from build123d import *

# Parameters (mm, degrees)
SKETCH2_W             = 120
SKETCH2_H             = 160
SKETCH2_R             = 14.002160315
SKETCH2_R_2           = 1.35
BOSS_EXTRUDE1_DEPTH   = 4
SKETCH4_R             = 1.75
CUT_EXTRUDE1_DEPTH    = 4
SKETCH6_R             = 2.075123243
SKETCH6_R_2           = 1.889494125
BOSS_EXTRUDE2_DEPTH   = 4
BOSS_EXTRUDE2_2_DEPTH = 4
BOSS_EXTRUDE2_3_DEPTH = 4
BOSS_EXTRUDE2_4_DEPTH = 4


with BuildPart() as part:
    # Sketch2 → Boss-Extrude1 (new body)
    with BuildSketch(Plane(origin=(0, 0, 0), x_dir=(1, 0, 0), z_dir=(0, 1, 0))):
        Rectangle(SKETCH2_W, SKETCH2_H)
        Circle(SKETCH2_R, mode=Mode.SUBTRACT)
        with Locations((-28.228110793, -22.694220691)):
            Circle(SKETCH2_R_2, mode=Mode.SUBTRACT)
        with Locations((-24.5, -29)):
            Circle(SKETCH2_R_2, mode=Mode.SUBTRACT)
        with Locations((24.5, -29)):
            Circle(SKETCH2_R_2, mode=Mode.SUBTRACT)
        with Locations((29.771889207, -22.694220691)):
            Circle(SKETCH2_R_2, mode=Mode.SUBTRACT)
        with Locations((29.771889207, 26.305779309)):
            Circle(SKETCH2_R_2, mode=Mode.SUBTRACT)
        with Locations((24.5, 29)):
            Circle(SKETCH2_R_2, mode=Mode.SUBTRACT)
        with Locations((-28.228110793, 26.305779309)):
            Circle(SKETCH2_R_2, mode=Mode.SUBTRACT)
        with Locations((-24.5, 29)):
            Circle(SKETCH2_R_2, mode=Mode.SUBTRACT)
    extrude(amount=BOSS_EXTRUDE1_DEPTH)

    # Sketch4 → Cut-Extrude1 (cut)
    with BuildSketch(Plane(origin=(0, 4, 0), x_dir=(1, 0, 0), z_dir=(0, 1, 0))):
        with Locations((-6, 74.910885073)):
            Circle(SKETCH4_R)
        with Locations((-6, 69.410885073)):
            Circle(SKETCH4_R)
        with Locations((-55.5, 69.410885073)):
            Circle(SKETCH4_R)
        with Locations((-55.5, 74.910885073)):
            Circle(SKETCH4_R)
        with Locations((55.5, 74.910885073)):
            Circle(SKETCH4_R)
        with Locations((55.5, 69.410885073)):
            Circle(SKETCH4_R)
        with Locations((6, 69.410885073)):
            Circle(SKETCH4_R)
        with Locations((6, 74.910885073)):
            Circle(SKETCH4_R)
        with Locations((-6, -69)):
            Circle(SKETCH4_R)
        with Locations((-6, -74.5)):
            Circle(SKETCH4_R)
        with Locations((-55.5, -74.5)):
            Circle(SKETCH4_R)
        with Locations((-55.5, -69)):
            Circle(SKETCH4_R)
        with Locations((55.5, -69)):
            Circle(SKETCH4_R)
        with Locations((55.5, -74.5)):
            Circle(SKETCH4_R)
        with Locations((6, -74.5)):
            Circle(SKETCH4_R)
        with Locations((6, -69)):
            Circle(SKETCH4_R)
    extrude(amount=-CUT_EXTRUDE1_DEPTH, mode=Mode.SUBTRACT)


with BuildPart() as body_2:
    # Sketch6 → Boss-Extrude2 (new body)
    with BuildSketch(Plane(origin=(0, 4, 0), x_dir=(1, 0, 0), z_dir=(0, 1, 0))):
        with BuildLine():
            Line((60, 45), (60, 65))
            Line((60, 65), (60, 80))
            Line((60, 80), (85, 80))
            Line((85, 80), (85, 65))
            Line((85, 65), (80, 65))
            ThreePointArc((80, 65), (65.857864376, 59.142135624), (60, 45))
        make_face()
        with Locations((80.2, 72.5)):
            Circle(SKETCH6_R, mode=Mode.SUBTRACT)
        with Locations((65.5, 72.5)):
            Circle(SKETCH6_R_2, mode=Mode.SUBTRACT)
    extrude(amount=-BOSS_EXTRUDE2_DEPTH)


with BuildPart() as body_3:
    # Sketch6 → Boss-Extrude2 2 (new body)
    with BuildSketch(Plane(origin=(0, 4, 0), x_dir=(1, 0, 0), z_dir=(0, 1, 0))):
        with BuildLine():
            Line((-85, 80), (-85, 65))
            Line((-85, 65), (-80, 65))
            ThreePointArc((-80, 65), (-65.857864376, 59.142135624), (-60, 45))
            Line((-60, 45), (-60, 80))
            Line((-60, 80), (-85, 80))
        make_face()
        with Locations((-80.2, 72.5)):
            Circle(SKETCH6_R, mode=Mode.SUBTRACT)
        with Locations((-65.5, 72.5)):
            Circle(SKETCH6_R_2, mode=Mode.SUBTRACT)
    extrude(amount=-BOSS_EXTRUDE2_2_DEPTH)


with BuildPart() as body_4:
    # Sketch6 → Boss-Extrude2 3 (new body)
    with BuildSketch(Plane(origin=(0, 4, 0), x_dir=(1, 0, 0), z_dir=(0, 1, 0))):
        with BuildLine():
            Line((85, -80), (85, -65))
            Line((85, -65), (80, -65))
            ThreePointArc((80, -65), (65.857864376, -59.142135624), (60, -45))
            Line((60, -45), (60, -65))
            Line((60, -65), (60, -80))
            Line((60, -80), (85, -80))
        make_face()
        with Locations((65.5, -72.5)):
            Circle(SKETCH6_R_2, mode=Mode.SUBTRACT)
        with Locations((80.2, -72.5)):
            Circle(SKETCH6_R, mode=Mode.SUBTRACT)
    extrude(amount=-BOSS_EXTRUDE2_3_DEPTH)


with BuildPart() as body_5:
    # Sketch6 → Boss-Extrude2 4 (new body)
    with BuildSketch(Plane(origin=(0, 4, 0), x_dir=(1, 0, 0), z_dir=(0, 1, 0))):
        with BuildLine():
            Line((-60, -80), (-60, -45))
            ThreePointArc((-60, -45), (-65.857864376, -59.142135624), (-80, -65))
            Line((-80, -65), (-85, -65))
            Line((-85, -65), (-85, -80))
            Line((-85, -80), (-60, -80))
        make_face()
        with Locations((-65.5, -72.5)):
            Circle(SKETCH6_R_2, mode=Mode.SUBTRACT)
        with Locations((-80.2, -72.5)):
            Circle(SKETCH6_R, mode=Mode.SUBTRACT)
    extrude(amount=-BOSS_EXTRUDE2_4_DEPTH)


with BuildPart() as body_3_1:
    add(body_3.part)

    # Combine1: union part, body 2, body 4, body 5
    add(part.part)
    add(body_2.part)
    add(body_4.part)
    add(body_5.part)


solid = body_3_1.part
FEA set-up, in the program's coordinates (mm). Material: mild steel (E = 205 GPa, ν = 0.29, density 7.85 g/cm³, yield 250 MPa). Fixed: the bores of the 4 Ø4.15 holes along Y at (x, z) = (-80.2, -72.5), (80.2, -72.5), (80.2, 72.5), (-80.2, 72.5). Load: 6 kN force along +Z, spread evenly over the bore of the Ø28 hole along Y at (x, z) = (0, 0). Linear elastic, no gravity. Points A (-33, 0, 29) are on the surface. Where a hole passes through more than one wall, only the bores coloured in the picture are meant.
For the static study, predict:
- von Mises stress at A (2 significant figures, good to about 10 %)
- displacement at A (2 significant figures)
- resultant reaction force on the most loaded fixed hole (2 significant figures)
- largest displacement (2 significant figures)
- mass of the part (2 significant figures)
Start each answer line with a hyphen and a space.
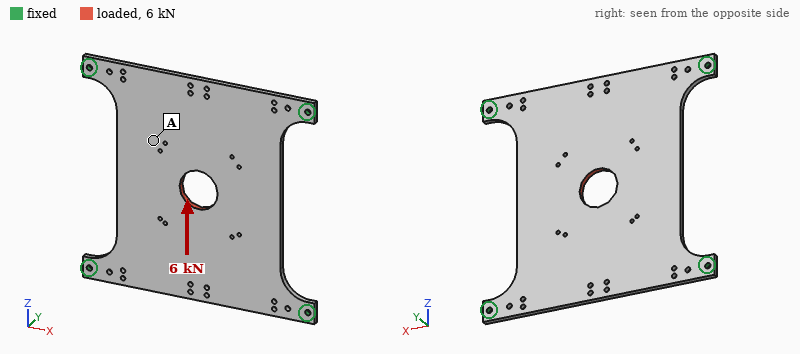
- 14 MPa
- 18 µm
- 2.0 kN
- 21 µm
- 630 g
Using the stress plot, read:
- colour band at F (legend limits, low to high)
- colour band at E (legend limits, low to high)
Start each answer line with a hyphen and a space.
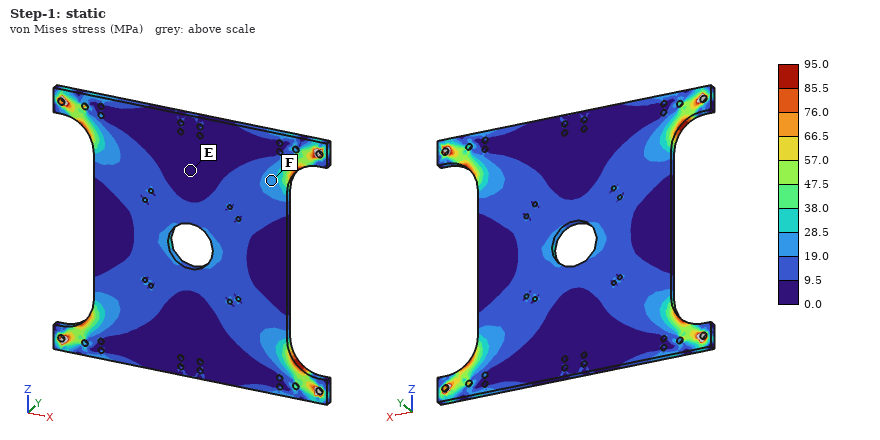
- 19.0 to 28.5 MPa
- 0.0 to 9.5 MPa
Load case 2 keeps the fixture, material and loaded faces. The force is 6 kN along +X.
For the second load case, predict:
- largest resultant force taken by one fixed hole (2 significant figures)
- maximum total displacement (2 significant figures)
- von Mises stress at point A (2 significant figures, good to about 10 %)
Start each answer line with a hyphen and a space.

- 1.6 kN
- 11 µm
- 13 MPa
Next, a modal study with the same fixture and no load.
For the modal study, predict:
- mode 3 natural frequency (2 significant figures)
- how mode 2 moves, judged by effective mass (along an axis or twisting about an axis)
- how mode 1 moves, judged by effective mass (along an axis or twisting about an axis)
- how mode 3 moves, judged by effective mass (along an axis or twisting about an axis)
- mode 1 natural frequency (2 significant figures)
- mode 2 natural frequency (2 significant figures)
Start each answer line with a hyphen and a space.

- 1000 Hz
- twisting about X
- along Y
- twisting about Z
- 450 Hz
- 820 Hz
